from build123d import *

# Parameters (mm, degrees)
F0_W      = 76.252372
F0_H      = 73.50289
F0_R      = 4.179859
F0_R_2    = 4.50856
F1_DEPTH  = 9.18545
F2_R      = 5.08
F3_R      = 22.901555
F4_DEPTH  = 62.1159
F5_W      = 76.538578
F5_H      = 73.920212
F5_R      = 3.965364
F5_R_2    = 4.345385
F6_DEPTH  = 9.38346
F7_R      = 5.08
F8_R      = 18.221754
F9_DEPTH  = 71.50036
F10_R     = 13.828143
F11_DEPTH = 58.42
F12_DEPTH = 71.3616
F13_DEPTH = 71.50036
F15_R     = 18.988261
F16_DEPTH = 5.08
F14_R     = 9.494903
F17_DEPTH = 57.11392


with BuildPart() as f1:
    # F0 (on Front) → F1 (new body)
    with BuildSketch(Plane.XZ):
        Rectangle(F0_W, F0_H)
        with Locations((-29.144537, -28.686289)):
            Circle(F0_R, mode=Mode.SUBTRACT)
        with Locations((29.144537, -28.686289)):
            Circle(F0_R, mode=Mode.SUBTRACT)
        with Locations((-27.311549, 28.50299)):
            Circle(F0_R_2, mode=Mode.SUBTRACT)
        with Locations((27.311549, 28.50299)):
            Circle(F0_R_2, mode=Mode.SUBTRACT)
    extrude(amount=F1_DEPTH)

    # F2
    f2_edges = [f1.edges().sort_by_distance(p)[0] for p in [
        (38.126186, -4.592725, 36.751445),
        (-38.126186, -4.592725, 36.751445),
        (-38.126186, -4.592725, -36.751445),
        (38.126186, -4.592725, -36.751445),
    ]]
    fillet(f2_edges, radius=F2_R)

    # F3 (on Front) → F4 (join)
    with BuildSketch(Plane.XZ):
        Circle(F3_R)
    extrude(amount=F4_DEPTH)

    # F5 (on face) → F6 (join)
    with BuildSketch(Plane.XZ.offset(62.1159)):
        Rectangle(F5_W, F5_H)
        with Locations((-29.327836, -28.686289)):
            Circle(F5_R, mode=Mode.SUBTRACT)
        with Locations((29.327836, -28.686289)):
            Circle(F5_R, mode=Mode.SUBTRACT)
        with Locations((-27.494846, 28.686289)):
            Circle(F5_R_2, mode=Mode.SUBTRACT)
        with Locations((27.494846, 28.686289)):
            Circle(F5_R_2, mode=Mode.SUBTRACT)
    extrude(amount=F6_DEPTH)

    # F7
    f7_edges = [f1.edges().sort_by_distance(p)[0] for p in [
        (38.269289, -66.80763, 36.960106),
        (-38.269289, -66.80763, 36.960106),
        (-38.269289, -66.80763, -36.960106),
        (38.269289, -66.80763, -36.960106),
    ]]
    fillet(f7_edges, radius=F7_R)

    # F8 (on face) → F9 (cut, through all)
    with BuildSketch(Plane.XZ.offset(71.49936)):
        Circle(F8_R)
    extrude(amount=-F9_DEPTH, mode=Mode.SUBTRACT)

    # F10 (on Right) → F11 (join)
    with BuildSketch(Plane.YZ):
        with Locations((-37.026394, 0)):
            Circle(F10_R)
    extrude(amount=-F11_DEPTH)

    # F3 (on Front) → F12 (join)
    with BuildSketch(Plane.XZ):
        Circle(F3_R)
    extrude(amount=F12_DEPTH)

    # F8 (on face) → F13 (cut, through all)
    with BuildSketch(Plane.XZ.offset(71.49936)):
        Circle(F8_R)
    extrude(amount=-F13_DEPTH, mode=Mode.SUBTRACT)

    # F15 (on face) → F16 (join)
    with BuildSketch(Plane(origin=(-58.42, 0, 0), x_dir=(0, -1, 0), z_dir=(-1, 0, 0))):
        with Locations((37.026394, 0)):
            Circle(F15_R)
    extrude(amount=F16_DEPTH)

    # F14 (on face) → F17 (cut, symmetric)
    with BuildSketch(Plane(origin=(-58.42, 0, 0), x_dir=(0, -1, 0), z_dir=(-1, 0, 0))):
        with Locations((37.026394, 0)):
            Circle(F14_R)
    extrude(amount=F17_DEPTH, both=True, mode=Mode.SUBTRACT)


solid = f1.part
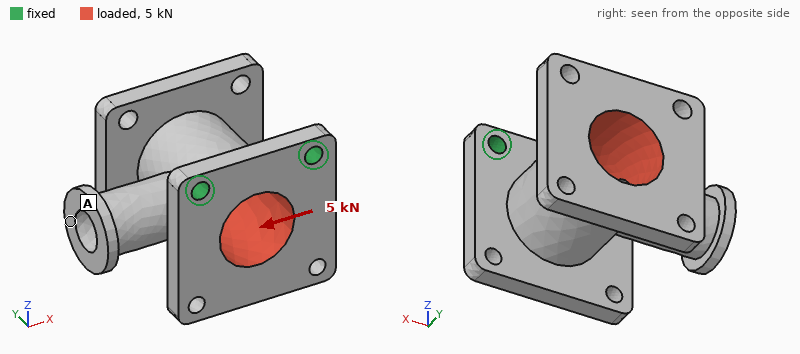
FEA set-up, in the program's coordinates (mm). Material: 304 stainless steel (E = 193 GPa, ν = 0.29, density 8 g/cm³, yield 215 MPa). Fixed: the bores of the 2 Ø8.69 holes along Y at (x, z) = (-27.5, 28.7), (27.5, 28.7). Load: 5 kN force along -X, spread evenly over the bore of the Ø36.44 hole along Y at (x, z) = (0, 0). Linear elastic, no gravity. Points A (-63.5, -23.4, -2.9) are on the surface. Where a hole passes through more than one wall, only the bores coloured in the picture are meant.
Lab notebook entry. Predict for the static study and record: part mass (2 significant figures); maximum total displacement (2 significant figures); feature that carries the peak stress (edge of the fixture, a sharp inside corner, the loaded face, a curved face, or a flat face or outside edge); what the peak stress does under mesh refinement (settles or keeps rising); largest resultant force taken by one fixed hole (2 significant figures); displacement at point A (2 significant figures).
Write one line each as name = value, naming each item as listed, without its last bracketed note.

part mass = 1.0 kg
maximum total displacement = 73 µm
feature that carries the peak stress = edge of the fixture
what the peak stress does under mesh refinement = keeps rising
largest resultant force taken by one fixed hole = 4.6 kN
displacement at point A = 70 µm
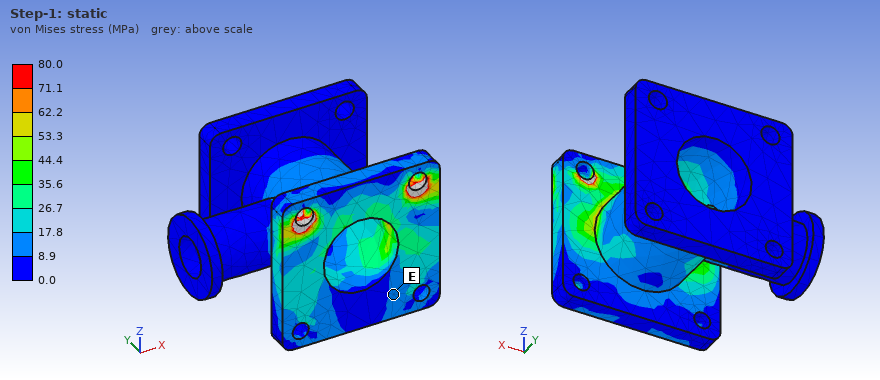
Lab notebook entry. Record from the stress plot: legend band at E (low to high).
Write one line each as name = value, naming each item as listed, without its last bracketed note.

legend band at E = 8.9 to 17.8 MPa
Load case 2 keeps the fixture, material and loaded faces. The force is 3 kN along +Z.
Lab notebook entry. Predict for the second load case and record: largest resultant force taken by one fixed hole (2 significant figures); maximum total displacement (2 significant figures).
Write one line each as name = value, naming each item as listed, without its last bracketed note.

largest resultant force taken by one fixed hole = 1.6 kN
maximum total displacement = 0.19 mm
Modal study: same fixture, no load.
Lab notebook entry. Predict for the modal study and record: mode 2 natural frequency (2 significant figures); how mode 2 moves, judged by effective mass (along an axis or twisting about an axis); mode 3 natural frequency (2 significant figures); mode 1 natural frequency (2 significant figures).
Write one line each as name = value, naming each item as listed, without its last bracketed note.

mode 2 natural frequency = 1400 Hz
how mode 2 moves, judged by effective mass = along X
mode 3 natural frequency = 2900 Hz
mode 1 natural frequency = 670 Hz
